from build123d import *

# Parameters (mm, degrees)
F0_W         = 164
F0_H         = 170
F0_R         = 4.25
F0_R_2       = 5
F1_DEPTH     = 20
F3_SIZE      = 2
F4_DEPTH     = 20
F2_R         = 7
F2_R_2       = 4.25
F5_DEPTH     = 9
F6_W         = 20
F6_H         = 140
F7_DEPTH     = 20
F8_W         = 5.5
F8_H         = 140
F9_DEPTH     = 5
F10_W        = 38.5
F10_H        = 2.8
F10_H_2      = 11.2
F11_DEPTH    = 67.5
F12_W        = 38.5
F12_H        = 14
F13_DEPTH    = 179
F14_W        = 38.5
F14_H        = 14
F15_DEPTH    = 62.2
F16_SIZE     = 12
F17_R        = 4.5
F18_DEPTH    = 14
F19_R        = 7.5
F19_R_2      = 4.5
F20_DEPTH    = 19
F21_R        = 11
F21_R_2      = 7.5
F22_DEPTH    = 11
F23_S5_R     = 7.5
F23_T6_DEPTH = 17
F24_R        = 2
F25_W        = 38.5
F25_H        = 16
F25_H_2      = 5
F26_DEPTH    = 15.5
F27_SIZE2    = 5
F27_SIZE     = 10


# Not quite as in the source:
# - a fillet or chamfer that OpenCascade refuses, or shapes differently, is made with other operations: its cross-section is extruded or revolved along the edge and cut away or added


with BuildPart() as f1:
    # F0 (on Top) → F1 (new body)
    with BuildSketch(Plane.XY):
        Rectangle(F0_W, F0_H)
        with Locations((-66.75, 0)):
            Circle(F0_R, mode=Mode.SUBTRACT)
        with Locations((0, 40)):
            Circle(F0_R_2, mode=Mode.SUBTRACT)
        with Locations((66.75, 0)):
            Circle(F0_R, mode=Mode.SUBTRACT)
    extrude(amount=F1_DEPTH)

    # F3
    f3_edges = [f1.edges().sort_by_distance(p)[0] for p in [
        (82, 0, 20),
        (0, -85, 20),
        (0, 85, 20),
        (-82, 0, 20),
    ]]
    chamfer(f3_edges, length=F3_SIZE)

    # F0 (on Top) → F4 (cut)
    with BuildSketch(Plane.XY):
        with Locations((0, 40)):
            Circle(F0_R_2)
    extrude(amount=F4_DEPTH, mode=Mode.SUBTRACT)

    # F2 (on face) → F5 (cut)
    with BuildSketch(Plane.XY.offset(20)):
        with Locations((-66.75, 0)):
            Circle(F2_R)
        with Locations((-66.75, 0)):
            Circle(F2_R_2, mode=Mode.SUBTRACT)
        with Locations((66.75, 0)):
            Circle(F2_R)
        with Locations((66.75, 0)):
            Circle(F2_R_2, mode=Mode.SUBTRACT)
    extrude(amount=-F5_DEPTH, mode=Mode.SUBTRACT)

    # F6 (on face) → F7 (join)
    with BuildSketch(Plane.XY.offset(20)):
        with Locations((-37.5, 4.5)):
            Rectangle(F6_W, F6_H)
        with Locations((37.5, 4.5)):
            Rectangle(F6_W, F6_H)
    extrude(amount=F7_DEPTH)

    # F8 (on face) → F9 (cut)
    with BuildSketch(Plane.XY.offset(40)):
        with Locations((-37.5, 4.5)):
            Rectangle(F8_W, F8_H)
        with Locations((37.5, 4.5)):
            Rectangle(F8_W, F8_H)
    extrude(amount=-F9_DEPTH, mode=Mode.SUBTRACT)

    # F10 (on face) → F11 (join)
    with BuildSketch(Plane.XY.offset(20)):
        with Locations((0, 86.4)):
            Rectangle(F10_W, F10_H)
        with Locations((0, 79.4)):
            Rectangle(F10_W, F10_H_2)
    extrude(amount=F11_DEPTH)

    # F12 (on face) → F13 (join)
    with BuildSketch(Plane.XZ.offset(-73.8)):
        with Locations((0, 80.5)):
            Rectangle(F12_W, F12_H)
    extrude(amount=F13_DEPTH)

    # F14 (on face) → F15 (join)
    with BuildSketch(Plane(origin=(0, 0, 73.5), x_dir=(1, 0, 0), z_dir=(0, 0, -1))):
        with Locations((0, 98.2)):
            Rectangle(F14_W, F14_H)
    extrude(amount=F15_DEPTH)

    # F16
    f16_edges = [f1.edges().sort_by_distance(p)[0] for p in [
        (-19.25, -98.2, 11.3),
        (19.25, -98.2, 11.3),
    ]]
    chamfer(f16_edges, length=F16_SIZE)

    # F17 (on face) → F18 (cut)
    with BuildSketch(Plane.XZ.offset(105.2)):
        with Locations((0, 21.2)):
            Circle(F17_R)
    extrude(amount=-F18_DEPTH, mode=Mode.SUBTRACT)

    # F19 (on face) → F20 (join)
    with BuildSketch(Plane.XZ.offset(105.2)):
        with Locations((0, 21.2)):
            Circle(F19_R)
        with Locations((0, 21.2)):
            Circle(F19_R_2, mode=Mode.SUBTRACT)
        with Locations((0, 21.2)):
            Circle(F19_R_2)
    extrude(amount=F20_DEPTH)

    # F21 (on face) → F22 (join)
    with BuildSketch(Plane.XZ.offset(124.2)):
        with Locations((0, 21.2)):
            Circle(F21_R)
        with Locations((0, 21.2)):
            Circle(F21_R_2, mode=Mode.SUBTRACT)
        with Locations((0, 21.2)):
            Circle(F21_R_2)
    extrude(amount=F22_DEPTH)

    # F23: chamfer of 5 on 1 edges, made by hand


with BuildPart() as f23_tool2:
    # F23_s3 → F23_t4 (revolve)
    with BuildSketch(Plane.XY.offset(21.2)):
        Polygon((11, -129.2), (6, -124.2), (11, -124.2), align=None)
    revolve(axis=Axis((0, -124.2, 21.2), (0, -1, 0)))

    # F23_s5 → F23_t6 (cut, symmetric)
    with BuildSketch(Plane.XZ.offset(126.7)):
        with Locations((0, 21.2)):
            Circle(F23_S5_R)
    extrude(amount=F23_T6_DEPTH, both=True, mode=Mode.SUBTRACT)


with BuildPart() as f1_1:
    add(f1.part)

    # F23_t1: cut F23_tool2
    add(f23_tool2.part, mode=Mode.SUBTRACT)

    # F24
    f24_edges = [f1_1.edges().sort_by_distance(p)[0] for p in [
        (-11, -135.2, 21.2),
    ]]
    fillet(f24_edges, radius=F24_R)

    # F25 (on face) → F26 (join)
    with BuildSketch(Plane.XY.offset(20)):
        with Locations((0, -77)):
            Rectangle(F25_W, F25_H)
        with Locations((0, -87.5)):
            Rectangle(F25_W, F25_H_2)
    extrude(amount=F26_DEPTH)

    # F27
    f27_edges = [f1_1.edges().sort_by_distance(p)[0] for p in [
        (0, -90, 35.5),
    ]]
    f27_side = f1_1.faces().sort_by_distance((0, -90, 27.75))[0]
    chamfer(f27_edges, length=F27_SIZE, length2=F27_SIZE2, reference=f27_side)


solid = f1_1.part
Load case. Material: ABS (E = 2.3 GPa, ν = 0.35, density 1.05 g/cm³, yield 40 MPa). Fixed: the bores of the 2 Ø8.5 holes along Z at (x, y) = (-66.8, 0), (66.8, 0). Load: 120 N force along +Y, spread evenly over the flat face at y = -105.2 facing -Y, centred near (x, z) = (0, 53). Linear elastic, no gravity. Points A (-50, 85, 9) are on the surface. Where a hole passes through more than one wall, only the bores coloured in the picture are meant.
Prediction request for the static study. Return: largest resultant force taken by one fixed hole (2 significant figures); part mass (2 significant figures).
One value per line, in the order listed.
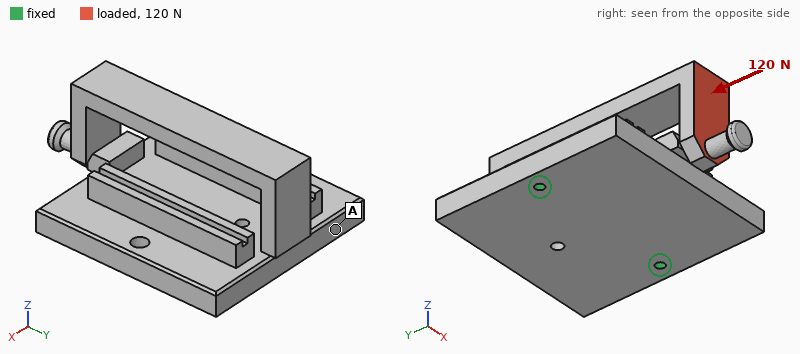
60 N
880 g
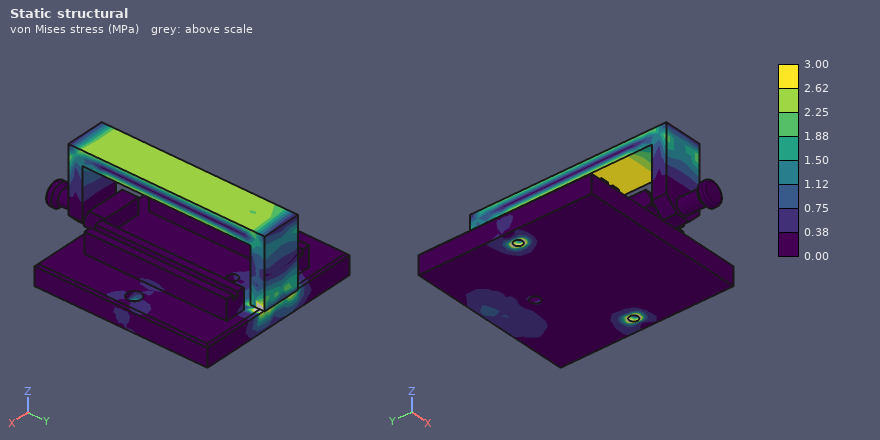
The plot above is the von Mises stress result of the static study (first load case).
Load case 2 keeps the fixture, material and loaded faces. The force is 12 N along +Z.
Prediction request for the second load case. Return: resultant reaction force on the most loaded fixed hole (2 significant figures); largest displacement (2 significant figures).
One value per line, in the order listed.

6.0 N
3.4 mm
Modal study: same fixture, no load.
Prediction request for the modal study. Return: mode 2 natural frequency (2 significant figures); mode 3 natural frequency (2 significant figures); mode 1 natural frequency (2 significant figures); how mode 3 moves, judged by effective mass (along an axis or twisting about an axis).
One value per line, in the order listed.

58 Hz
150 Hz
39 Hz
along Y
